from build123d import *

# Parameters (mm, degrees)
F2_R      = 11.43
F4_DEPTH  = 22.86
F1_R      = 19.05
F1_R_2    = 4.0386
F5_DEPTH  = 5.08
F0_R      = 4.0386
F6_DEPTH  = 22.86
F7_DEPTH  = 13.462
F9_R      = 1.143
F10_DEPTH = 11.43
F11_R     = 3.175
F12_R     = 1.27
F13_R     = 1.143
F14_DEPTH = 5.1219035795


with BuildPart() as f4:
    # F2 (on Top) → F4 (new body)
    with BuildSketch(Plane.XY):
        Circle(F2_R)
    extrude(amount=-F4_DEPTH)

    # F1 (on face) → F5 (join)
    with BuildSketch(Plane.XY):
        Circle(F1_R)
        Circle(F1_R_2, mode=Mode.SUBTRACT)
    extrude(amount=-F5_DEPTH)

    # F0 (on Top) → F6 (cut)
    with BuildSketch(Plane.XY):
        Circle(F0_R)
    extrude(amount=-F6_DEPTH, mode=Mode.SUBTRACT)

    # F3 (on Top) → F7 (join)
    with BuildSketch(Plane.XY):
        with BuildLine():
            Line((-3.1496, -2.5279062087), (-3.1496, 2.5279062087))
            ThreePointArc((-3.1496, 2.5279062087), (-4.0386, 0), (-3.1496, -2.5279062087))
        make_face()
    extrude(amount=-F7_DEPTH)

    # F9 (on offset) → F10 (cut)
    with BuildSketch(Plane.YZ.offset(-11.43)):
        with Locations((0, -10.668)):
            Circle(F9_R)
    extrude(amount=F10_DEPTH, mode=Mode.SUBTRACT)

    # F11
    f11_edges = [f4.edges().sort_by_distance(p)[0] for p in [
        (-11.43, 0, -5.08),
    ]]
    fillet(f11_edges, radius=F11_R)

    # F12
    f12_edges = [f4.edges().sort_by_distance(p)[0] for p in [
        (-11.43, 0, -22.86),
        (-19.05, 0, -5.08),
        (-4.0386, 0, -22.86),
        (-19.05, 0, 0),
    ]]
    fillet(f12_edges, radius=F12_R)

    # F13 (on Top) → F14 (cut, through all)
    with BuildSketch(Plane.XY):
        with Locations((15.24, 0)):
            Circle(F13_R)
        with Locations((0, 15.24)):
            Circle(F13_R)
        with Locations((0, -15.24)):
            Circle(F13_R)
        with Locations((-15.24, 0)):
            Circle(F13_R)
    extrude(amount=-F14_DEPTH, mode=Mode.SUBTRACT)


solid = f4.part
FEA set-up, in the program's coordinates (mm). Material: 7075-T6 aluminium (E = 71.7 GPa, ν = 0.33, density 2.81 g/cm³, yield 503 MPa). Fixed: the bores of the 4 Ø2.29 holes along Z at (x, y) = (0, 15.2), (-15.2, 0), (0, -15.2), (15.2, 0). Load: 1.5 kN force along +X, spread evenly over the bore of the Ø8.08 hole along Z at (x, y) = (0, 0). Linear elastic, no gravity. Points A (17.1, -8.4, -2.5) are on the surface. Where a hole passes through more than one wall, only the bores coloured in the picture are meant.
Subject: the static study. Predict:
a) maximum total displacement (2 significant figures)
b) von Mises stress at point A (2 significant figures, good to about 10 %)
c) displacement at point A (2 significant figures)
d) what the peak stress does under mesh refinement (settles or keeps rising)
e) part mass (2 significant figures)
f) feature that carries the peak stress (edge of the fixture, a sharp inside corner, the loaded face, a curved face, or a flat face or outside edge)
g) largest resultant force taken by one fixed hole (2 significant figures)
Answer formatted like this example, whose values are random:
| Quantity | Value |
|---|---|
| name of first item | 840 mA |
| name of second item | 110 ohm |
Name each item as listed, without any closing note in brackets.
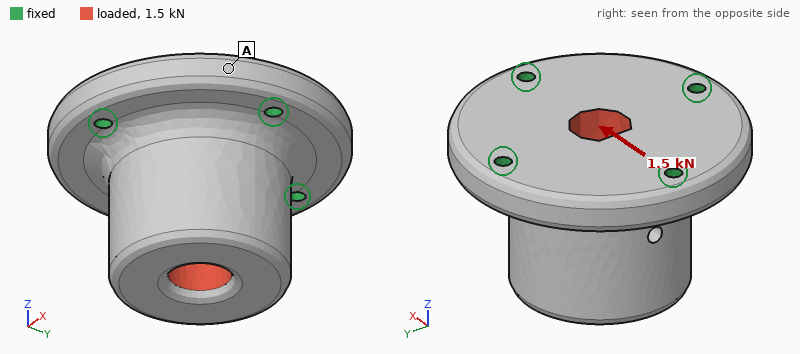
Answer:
| Quantity | Value |
|---|---|
| maximum total displacement | 6.1 µm |
| von Mises stress at point A | 4.7 MPa |
| displacement at point A | 1.6 µm |
| what the peak stress does under mesh refinement | keeps rising |
| part mass | 33 g |
| feature that carries the peak stress | edge of the fixture |
| largest resultant force taken by one fixed hole | 680 N |
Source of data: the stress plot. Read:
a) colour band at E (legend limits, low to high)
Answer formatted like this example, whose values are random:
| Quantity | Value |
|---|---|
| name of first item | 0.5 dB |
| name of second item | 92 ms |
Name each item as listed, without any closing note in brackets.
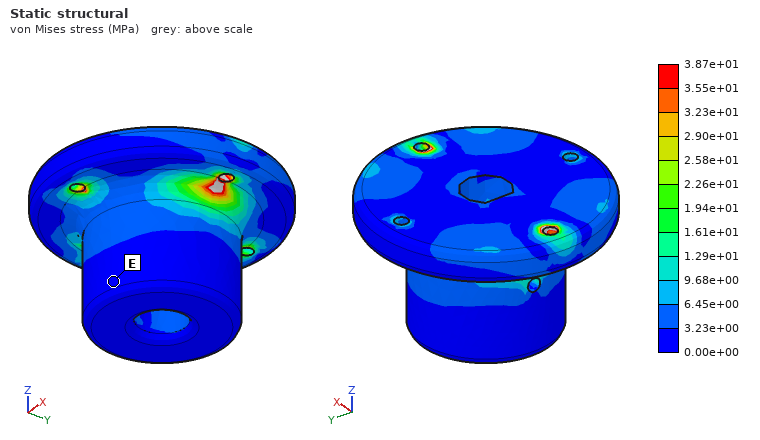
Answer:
| Quantity | Value |
|---|---|
| colour band at E | 0.00e+00 to 3.23e+00 MPa |
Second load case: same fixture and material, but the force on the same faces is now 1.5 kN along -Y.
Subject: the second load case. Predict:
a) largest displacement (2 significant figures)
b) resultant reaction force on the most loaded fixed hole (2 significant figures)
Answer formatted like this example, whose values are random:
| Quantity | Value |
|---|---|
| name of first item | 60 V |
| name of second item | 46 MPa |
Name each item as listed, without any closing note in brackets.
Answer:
| Quantity | Value |
|---|---|
| largest displacement | 6.1 µm |
| resultant reaction force on the most loaded fixed hole | 660 N |
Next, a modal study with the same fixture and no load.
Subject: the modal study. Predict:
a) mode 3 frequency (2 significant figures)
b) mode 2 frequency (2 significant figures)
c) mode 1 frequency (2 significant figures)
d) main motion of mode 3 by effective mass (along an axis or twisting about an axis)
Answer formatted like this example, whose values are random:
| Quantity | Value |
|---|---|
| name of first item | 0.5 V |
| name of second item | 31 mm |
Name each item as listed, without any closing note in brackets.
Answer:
| Quantity | Value |
|---|---|
| mode 3 frequency | 25 kHz |
| mode 2 frequency | 19 kHz |
| mode 1 frequency | 19 kHz |
| main motion of mode 3 by effective mass | along Z |
